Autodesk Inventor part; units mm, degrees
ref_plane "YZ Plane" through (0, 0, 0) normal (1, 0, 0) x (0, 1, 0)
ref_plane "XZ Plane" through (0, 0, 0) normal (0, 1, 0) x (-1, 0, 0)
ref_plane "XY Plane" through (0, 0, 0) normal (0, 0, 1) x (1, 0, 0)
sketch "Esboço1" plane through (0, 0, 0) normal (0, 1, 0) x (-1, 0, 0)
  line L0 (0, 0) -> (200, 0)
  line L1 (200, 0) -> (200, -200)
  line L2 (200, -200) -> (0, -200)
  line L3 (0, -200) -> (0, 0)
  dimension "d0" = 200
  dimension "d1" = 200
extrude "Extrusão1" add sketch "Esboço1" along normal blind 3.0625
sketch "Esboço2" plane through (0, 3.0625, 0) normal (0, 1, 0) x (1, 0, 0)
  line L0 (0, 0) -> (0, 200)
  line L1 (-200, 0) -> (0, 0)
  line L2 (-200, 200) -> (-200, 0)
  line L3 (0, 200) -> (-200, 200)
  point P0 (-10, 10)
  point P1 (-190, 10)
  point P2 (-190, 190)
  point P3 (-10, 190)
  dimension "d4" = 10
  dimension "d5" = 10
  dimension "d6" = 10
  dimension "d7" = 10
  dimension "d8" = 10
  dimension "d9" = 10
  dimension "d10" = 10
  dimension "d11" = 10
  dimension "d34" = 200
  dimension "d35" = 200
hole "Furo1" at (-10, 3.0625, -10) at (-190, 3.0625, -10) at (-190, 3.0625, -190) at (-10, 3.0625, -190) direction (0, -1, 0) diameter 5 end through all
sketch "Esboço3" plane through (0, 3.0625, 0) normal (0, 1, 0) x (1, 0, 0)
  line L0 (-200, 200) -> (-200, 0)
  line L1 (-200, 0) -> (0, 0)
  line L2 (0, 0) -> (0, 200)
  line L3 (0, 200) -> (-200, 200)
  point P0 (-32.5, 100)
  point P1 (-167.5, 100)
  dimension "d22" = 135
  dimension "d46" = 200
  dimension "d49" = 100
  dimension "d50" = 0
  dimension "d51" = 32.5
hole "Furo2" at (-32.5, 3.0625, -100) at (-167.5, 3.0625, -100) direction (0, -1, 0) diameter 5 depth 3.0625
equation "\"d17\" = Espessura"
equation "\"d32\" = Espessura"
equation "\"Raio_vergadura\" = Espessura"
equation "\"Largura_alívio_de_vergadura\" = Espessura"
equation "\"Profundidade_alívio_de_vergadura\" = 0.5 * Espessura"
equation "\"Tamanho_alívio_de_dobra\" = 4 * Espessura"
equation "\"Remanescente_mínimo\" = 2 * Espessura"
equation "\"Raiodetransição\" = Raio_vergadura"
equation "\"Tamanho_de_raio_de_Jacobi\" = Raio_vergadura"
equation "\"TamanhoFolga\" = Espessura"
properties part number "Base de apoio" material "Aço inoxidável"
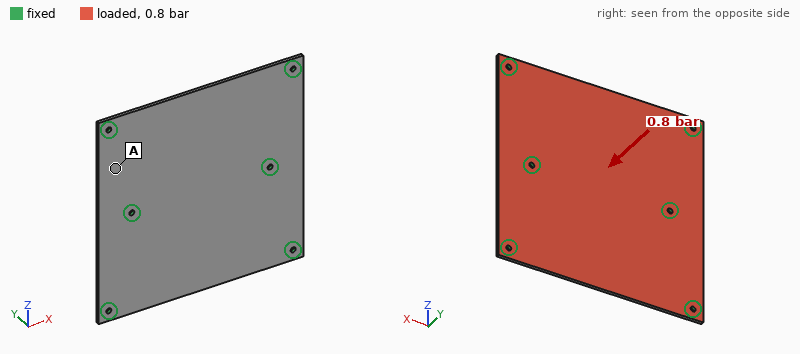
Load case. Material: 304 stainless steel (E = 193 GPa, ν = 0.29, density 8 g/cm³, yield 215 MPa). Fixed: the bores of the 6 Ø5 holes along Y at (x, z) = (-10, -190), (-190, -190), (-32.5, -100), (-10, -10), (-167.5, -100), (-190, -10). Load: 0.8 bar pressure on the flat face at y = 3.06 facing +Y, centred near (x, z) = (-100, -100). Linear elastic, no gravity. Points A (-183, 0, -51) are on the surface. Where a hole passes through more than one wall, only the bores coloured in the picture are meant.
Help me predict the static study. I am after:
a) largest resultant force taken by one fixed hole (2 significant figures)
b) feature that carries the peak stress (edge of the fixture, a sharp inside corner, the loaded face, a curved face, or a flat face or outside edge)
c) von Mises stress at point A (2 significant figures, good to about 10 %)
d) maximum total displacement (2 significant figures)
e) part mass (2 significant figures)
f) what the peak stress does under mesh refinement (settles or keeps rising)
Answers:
870 N
edge of the fixture
28 MPa
0.50 mm
980 g
keeps rising
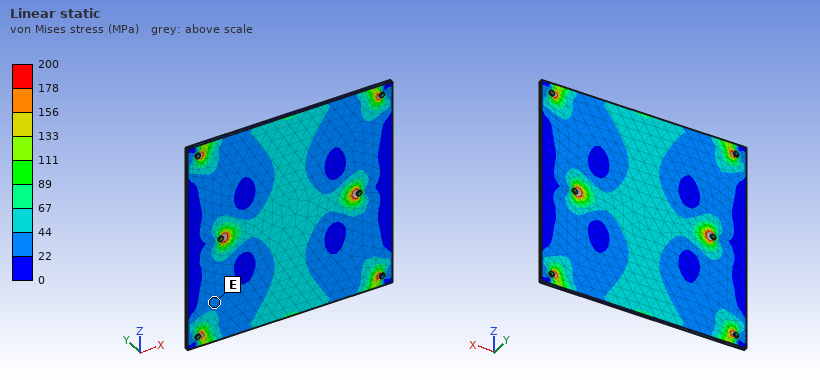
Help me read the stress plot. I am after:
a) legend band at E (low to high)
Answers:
22 to 44 MPa
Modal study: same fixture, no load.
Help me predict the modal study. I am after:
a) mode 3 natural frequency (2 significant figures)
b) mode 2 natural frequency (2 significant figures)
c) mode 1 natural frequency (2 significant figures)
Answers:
1000 Hz
530 Hz
510 Hz
